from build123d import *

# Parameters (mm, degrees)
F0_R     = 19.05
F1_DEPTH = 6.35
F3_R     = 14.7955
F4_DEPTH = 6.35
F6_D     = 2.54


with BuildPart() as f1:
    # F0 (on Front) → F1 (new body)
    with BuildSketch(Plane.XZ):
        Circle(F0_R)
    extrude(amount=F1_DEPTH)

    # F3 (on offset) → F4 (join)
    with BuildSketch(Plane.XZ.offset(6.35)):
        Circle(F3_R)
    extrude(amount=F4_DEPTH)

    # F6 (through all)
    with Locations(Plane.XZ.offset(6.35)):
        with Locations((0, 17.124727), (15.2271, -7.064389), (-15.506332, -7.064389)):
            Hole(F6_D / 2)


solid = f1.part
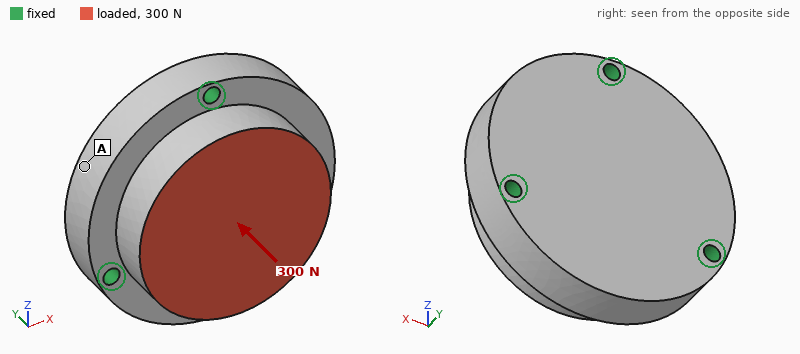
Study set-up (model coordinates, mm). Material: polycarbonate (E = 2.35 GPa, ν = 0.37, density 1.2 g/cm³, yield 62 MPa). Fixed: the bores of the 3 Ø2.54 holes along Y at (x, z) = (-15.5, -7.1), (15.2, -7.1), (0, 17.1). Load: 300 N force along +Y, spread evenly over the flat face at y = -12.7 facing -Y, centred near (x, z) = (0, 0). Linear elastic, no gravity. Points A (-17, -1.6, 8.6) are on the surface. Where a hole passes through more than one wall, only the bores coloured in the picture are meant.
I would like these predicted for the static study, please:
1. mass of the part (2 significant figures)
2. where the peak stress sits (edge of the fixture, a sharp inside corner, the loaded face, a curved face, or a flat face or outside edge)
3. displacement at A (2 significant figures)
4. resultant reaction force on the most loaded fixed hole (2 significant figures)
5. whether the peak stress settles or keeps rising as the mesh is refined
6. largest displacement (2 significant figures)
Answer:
14 g
edge of the fixture
14 µm
110 N
keeps rising
20 µm
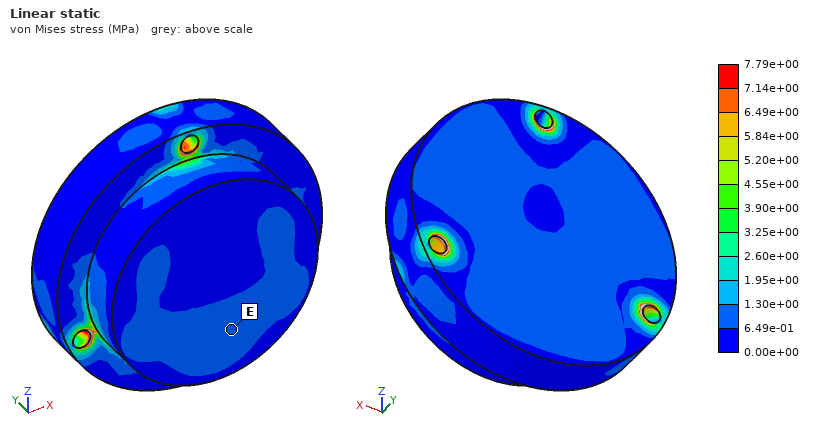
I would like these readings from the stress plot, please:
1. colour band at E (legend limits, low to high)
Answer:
6.49e-01 to 1.30e+00 MPa
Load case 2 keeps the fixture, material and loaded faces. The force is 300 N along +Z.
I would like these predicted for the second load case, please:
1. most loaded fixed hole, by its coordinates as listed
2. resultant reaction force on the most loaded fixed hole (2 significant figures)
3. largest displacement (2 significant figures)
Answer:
(0, 17.1)
170 N
35 µm
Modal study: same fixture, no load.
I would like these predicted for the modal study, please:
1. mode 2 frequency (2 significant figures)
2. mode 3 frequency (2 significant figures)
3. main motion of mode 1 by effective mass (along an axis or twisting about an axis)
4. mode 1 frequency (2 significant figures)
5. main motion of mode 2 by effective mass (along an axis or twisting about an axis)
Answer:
6900 Hz
7500 Hz
along Y
6100 Hz
along Y
